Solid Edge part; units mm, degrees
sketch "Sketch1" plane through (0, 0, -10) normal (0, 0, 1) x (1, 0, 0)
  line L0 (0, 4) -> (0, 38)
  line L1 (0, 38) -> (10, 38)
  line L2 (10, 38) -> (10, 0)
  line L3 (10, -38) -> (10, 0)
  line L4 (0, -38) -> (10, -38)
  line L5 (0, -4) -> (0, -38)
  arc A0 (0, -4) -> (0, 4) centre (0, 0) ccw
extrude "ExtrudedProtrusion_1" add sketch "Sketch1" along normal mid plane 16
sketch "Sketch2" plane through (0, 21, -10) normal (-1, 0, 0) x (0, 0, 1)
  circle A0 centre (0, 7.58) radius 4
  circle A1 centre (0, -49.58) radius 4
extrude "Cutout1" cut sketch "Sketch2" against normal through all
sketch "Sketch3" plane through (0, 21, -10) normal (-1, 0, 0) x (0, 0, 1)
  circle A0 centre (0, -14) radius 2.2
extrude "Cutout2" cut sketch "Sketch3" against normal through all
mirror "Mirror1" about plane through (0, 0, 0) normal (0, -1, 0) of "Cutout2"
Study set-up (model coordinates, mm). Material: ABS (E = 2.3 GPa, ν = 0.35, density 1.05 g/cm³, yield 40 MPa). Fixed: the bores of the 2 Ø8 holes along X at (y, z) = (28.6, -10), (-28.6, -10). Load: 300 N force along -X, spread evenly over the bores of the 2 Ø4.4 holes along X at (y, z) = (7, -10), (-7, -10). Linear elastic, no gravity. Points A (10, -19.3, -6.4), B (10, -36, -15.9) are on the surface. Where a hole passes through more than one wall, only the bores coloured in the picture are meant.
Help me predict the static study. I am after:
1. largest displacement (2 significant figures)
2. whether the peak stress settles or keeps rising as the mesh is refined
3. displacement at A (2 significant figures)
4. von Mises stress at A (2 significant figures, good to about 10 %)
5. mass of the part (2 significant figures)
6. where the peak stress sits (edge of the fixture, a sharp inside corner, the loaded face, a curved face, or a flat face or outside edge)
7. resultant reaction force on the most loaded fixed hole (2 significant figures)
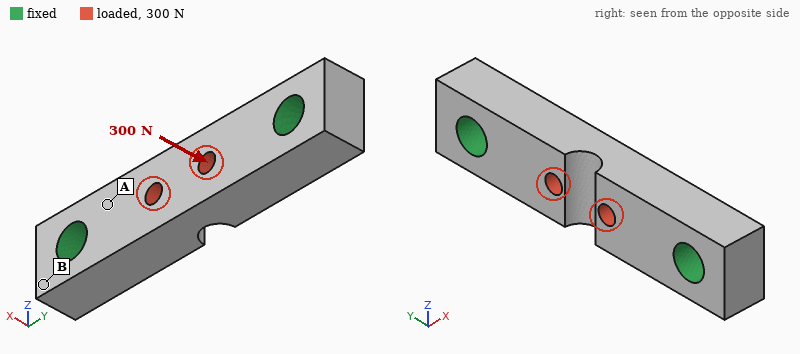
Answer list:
0.12 mm
keeps rising
0.029 mm
3.8 MPa
11 g
edge of the fixture
170 N
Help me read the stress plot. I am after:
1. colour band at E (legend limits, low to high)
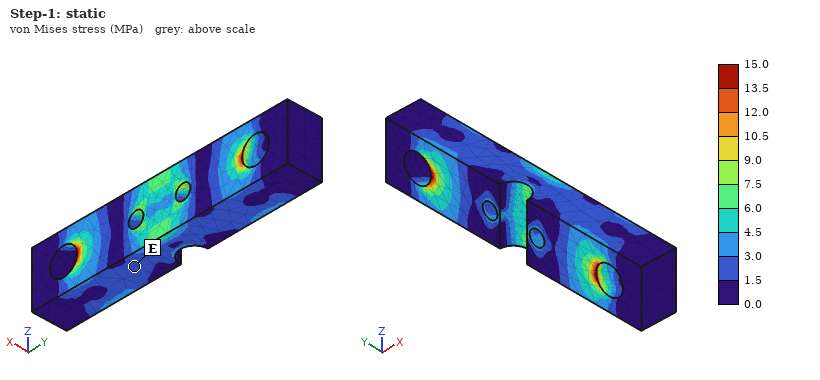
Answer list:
1.5 to 3.0 MPa
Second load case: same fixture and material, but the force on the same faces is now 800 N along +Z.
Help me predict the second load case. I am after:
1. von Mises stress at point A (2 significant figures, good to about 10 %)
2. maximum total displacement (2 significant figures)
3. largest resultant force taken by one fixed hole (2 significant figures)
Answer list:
5.9 MPa
0.19 mm
400 N
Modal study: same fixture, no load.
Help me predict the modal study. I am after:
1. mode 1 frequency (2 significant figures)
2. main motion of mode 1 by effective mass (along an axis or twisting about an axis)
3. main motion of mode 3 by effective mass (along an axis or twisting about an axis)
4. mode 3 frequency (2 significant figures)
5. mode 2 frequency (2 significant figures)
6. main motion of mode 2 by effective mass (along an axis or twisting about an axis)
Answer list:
4400 Hz
along X
twisting about Y
7700 Hz
5400 Hz
along Z
